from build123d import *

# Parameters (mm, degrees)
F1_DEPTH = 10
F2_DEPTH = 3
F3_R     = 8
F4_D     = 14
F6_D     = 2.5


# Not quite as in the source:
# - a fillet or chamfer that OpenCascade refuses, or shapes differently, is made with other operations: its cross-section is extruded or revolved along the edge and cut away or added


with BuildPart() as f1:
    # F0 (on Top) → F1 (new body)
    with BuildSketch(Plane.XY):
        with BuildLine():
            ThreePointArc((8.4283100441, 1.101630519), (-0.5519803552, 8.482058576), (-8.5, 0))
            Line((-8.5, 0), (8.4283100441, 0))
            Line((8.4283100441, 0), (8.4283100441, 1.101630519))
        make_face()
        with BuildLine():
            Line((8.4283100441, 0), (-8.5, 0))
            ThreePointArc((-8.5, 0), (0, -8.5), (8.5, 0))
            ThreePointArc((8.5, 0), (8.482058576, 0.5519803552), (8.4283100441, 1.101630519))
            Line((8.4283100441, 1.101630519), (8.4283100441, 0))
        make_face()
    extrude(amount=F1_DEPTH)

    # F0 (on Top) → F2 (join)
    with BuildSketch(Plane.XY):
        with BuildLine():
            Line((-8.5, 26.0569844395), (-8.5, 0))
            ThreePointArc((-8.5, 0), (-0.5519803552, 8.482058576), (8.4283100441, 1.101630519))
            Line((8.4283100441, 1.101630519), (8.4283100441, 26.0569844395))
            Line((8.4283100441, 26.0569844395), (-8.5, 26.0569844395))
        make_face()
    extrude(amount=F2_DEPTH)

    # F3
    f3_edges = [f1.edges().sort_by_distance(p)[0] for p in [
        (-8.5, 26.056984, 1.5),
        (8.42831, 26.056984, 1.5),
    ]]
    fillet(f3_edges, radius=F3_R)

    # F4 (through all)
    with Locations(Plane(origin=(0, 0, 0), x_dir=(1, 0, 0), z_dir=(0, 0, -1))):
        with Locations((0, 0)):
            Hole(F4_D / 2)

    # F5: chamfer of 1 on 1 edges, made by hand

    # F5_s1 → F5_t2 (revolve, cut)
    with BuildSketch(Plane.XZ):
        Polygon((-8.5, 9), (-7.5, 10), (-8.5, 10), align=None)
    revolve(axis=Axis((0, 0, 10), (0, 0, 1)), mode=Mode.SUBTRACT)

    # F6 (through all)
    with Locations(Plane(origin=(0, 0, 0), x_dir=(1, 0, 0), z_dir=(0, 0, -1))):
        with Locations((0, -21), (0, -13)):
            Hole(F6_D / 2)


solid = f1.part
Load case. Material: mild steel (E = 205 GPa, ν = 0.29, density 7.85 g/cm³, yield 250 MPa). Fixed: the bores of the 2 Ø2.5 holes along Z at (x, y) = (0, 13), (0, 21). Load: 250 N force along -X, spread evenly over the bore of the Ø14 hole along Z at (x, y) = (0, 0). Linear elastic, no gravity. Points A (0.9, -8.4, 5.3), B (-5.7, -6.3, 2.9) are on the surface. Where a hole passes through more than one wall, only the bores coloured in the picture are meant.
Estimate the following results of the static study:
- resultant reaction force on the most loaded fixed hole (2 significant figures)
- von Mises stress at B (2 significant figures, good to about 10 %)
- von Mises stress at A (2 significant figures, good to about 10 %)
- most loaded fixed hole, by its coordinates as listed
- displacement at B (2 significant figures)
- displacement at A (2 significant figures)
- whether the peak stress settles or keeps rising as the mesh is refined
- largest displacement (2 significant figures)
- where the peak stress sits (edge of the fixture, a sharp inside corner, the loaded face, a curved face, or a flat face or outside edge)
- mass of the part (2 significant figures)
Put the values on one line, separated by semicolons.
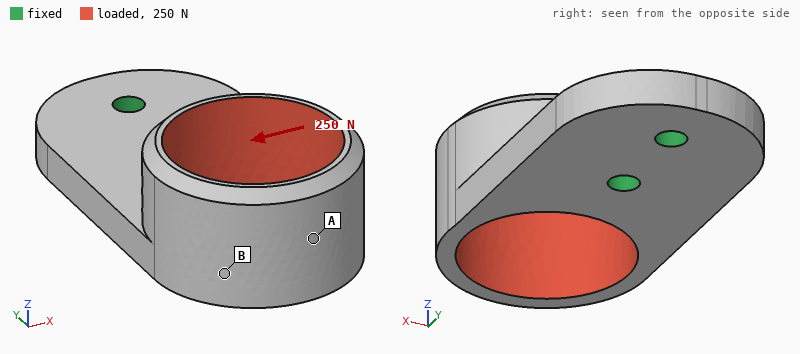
540 N; 36 MPa; 11 MPa; (0, 13); 20 µm; 20 µm; keeps rising; 23 µm; edge of the fixture; 12 g
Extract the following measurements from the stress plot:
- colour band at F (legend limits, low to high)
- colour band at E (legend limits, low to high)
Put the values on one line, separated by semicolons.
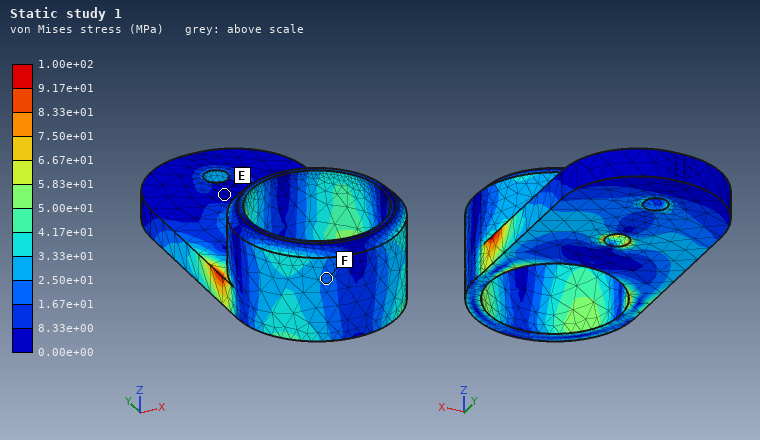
1.67e+01 to 2.50e+01 MPa; 0.00e+00 to 8.33e+00 MPa
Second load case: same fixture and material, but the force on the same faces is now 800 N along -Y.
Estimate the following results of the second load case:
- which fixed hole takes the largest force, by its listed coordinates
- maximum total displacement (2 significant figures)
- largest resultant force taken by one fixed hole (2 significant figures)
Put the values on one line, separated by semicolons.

(0, 13); 85 µm; 530 N
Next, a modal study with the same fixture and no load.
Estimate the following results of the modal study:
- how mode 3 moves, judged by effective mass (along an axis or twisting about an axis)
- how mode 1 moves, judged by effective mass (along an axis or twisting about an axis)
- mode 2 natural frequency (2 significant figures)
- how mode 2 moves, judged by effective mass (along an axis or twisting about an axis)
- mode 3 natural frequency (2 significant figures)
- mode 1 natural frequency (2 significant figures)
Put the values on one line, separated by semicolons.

twisting about Y; along Z; 8100 Hz; along X; 10 kHz; 4800 Hz
